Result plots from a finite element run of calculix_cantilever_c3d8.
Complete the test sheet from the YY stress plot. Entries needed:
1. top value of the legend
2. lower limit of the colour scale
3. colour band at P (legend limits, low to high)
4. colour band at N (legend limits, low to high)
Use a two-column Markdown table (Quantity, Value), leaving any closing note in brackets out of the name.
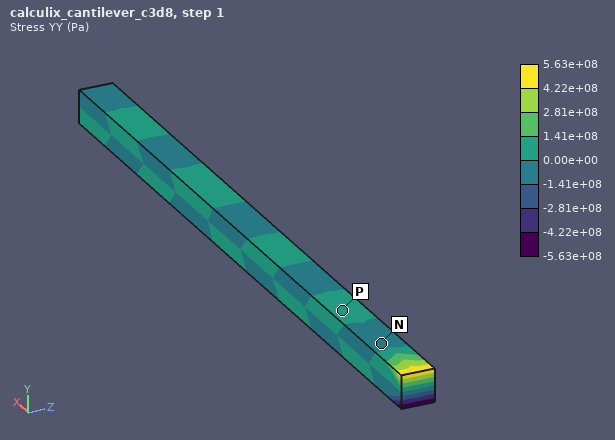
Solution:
| Quantity | Value |
|---|---|
| top value of the legend | 5.63e+08 Pa |
| lower limit of the colour scale | -5.63e+08 Pa |
| colour band at P | 0.00e+00 to 1.41e+08 Pa |
| colour band at N | -1.41e+08 to 0.00e+00 Pa |
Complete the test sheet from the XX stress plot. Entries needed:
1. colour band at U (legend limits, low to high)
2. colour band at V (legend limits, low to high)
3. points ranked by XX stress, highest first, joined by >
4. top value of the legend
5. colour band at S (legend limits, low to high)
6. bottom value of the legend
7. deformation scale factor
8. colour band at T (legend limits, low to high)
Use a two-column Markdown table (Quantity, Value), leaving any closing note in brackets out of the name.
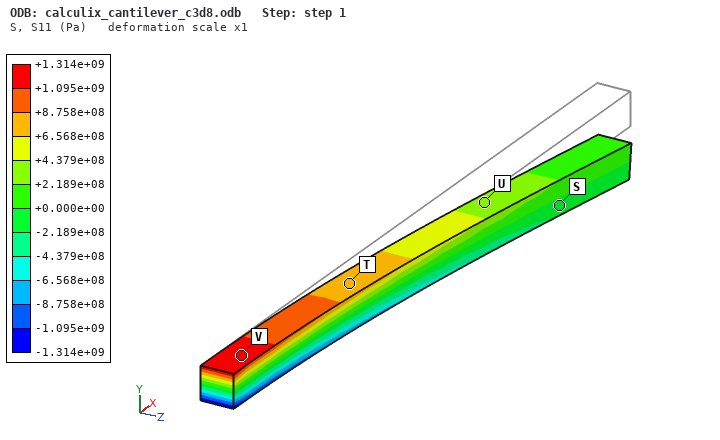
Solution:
| Quantity | Value |
|---|---|
| colour band at U | +2.189e+08 to +4.379e+08 Pa |
| colour band at V | +1.095e+09 to +1.314e+09 Pa |
| points ranked by XX stress, highest first, joined by > | V > T > U > S |
| top value of the legend | +1.314e+09 Pa |
| colour band at S | -2.189e+08 to +0.000e+00 Pa |
| bottom value of the legend | -1.314e+09 Pa |
| deformation scale factor | 1 |
| colour band at T | +6.568e+08 to +8.758e+08 Pa |
